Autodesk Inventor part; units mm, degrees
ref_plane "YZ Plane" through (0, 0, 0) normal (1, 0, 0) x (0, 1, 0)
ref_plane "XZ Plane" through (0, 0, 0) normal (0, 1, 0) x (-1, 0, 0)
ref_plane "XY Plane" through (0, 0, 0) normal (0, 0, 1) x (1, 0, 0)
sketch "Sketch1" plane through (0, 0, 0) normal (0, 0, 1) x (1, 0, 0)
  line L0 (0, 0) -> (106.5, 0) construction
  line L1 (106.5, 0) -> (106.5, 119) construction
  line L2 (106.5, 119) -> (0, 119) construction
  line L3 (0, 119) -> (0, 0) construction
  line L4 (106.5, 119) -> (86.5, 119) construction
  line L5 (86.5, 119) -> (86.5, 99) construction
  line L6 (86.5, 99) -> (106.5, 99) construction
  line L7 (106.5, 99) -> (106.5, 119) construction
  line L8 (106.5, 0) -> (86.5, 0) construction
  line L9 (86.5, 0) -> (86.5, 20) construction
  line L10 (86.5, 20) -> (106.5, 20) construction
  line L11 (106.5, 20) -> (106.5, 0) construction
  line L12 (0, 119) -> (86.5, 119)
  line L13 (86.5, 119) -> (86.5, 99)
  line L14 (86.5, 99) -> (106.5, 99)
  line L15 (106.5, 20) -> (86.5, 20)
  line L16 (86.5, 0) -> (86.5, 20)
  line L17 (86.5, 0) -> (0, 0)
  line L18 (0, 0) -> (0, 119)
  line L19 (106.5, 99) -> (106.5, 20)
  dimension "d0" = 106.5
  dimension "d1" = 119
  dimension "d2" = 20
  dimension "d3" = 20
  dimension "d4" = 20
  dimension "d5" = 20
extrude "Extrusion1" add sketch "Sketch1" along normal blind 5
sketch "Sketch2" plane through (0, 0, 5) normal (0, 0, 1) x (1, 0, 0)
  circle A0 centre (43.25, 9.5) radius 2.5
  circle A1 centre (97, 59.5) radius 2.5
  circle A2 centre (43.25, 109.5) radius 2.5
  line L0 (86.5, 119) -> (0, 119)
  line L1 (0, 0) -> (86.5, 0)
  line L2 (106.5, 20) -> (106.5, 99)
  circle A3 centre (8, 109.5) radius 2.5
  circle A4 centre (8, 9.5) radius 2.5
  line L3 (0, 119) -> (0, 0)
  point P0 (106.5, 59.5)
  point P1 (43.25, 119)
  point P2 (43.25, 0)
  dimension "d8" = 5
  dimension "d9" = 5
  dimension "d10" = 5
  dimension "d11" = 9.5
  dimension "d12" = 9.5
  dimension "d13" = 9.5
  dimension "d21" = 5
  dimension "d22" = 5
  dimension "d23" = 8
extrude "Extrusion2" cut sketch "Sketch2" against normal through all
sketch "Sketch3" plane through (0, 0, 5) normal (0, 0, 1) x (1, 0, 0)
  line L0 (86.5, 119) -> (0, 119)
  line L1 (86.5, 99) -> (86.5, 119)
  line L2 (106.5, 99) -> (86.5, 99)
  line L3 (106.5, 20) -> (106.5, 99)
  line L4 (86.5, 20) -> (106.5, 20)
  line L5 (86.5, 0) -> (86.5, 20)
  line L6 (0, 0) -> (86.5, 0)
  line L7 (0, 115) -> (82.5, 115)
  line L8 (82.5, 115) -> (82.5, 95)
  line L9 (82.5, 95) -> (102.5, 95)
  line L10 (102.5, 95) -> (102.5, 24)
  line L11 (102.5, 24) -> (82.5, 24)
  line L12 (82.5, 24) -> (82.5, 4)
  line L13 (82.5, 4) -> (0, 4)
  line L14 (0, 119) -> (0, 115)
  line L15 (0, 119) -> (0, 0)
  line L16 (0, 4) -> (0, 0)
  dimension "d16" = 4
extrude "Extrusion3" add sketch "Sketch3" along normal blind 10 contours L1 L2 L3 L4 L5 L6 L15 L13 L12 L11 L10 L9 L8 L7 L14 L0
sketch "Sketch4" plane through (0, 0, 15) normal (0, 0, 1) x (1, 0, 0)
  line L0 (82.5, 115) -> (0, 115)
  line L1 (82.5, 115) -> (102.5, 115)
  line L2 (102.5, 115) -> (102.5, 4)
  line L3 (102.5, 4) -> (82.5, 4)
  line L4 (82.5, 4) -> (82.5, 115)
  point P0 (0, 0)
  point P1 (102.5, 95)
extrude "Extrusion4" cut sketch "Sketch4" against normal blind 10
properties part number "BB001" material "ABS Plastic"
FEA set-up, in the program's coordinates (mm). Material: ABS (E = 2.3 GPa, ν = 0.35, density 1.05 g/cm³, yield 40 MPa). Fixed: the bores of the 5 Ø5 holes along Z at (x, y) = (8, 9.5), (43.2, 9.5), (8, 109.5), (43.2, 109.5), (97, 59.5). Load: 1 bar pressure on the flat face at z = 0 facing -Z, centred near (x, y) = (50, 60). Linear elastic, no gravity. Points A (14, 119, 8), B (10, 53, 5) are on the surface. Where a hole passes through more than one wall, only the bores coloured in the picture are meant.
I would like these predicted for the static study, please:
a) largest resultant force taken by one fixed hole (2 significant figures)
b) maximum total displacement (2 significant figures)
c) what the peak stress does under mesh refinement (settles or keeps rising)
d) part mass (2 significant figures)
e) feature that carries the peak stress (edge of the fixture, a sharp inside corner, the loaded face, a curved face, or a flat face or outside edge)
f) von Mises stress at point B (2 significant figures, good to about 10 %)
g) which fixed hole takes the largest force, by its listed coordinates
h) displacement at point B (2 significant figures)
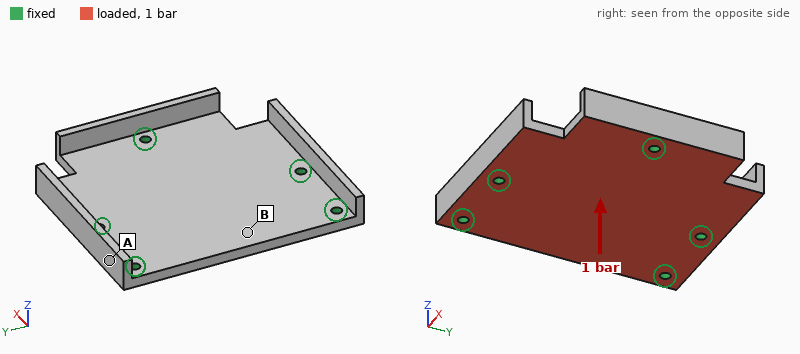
330 N
1.2 mm
keeps rising
72 g
edge of the fixture
9.1 MPa
(97, 59.5)
1.1 mm
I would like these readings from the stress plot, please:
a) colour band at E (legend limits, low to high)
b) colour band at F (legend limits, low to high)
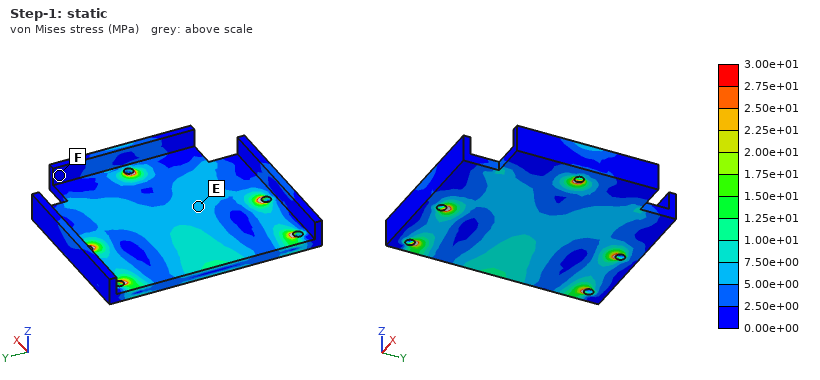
5.00e+00 to 7.50e+00 MPa
0.00e+00 to 2.50e+00 MPa
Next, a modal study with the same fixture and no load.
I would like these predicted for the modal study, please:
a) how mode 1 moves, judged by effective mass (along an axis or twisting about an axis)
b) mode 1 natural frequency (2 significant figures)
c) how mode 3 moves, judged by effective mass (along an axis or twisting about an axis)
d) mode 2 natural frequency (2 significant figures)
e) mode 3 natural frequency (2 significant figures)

along Z
800 Hz
along Z
1000 Hz
1200 Hz
